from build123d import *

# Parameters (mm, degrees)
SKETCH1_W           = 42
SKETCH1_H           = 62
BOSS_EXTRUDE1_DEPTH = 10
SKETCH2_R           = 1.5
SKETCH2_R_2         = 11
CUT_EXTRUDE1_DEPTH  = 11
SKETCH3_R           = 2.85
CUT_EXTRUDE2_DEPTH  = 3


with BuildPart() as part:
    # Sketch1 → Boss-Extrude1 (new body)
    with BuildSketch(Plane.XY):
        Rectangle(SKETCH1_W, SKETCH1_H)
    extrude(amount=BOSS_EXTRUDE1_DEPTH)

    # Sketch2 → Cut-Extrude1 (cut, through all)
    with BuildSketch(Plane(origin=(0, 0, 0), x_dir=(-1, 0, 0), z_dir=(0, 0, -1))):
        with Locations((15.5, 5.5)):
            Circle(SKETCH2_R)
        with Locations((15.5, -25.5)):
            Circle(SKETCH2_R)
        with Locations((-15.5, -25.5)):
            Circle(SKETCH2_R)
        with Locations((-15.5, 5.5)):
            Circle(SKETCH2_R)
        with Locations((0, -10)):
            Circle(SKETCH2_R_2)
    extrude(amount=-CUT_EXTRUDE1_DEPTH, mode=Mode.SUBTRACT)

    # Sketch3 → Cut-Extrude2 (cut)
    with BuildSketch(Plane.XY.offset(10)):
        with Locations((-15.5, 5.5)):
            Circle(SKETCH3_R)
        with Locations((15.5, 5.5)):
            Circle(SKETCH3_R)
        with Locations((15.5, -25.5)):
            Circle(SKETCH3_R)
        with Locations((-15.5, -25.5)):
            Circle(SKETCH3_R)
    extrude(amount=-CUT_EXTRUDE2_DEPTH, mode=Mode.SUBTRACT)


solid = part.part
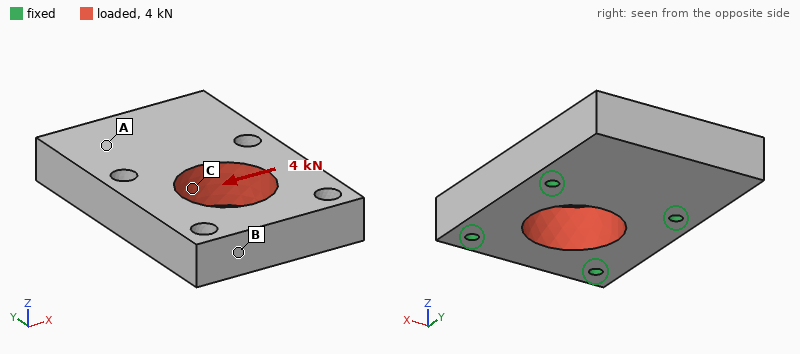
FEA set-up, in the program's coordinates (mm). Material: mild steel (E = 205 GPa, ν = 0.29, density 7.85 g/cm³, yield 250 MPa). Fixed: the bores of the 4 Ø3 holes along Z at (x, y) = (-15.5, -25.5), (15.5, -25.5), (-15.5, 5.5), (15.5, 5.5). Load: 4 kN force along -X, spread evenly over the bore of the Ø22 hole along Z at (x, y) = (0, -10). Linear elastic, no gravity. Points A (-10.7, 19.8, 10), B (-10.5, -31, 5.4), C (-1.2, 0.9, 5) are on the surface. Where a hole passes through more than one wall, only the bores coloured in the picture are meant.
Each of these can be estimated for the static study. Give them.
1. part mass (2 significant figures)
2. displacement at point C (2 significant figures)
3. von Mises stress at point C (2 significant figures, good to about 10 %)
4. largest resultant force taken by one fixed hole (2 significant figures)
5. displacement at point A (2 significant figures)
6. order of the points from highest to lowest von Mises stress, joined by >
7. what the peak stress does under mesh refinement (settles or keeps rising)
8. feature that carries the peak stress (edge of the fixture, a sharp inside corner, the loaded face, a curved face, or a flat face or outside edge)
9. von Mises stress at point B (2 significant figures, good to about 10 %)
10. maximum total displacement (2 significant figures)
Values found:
170 g
0.67 µm
10 MPa
1.0 kN
0.23 µm
C > B > A
keeps rising
edge of the fixture
5.7 MPa
1.5 µm
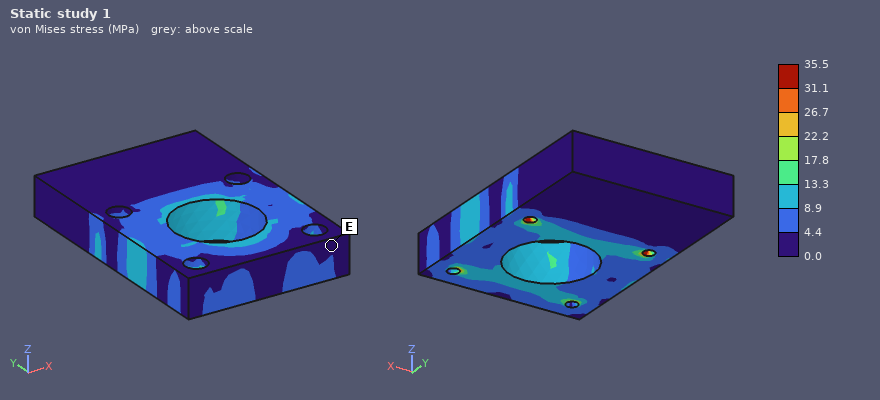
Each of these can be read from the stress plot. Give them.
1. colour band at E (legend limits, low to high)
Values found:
0.0 to 4.4 MPa
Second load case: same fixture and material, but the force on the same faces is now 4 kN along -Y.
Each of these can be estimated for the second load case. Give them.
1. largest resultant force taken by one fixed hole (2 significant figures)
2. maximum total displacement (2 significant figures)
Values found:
1.0 kN
1.6 µm
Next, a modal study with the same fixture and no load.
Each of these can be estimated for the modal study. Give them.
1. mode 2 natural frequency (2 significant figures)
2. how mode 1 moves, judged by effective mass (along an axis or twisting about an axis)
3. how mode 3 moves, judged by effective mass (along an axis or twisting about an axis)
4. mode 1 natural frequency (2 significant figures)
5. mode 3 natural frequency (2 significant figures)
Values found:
16 kHz
along Z
along X
7700 Hz
21 kHz
